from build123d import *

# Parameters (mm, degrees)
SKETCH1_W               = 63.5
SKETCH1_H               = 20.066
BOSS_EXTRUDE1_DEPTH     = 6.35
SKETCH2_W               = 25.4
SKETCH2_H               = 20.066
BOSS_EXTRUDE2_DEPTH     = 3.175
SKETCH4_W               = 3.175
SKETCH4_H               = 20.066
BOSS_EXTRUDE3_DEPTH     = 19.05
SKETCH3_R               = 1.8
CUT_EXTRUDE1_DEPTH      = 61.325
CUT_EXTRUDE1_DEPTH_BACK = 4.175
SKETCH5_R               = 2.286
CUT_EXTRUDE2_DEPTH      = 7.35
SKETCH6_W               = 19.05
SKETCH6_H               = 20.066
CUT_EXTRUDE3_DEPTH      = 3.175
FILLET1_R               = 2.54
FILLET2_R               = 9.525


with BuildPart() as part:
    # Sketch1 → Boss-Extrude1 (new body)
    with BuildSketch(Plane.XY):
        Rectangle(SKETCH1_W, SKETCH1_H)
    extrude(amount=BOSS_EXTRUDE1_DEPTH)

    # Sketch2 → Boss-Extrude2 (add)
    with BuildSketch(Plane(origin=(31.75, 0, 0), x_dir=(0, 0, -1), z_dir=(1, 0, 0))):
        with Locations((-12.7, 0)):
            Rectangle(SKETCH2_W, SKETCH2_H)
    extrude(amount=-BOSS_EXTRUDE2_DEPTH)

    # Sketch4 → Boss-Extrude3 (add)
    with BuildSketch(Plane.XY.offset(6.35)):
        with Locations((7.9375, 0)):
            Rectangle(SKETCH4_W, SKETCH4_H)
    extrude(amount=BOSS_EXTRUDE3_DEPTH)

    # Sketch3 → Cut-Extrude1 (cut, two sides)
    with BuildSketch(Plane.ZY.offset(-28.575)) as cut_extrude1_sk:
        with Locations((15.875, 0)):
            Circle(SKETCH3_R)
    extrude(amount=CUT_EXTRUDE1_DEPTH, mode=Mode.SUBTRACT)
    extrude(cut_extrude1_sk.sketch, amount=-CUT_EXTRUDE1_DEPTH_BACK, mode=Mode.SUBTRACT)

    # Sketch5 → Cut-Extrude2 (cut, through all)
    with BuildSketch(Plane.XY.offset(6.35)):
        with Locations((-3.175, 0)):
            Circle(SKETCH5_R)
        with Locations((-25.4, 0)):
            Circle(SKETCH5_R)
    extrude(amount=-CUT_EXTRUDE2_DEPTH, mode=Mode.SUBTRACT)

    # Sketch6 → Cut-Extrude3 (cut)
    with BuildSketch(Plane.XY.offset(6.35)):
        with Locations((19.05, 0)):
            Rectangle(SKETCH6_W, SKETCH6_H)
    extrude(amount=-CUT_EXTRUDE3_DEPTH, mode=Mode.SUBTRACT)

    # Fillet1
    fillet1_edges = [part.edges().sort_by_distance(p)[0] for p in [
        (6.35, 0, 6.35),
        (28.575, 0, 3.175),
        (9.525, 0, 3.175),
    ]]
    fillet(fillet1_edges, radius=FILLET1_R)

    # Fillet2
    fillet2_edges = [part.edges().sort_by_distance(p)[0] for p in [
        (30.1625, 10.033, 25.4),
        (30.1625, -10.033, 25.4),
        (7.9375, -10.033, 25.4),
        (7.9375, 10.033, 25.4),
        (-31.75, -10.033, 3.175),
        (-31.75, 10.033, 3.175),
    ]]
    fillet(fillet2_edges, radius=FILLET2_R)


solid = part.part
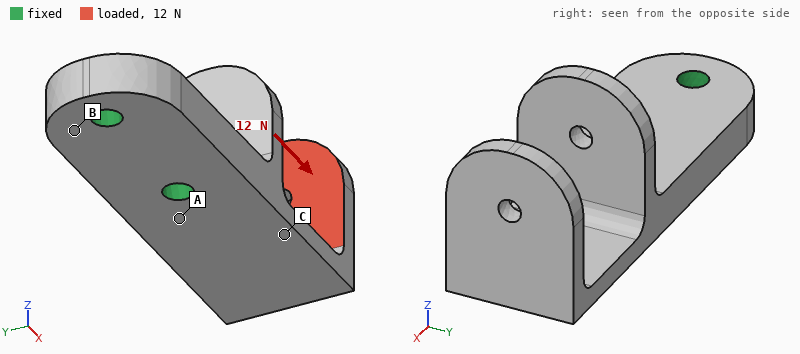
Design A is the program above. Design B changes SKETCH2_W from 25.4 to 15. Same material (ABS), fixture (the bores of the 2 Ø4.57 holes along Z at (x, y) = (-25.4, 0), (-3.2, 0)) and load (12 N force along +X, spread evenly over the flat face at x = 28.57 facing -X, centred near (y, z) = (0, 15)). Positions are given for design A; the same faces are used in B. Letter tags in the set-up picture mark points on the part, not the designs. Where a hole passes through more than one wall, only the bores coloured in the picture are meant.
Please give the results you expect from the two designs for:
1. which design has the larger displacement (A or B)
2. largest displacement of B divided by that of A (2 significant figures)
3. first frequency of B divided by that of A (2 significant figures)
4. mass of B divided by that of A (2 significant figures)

A
0.63
1.2
0.96
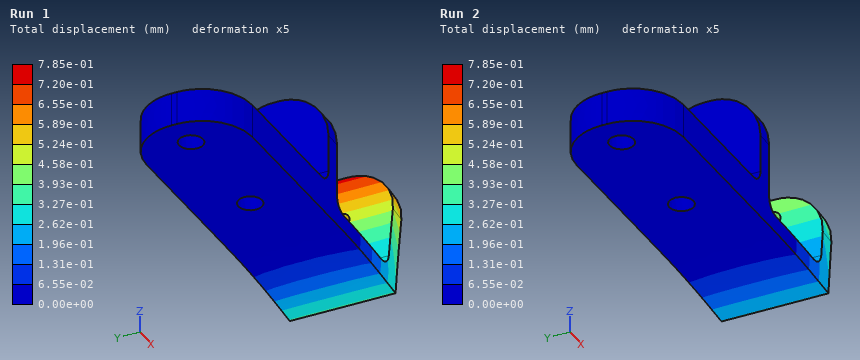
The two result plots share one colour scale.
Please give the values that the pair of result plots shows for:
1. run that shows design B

Run 2
